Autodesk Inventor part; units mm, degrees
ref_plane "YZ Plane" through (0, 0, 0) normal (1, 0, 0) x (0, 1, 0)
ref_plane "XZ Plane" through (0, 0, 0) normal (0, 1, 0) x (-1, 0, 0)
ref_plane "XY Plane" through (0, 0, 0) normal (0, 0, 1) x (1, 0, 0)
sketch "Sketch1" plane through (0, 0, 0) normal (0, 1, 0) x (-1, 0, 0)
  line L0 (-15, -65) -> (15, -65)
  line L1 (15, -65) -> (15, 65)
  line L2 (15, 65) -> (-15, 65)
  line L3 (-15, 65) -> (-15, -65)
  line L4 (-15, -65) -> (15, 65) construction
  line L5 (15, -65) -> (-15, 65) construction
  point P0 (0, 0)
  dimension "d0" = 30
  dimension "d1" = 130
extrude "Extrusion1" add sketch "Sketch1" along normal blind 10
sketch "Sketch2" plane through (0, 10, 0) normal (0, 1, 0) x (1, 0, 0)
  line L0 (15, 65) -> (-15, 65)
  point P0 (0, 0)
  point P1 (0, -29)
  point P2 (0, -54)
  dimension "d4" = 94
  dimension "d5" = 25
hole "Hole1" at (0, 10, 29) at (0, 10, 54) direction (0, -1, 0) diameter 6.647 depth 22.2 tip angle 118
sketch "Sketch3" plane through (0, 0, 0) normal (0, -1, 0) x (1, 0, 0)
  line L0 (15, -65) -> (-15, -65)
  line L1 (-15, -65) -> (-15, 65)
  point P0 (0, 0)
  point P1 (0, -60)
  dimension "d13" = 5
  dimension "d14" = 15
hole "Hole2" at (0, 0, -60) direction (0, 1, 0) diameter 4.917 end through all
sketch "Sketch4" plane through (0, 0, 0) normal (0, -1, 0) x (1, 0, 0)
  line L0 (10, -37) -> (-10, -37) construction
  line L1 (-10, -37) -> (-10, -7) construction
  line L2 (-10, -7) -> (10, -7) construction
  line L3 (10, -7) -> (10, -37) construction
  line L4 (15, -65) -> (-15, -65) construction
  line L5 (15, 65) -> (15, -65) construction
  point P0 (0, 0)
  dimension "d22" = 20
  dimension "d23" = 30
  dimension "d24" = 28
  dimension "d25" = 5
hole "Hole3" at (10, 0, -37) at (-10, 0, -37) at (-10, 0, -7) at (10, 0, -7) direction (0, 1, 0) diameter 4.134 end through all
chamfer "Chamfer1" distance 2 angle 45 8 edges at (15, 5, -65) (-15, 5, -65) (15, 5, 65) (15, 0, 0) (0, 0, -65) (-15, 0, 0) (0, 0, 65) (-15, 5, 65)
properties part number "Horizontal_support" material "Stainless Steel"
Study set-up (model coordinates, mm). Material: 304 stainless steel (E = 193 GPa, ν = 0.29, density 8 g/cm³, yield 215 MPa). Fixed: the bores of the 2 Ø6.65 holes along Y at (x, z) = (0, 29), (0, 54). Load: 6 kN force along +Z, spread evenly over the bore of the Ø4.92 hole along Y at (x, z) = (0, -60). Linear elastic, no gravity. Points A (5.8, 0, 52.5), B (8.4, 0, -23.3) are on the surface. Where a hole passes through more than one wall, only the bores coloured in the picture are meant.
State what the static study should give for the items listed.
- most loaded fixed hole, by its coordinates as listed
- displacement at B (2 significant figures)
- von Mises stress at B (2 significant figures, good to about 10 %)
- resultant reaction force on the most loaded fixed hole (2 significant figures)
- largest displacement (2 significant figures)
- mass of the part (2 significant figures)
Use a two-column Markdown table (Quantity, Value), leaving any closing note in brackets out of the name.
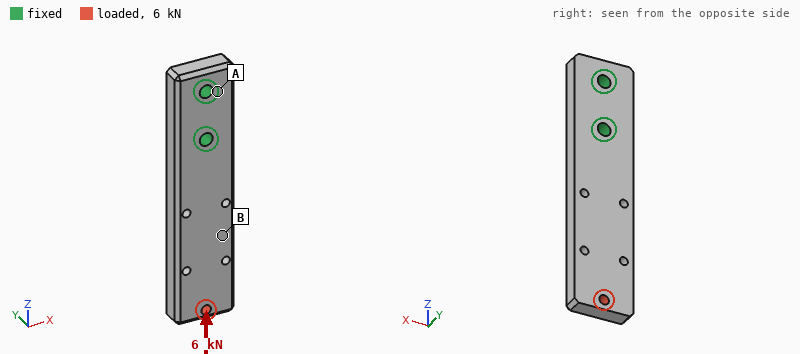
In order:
| Quantity | Value |
|---|---|
| most loaded fixed hole, by its coordinates as listed | (0, 29) |
| displacement at B | 6.5 µm |
| von Mises stress at B | 20 MPa |
| resultant reaction force on the most loaded fixed hole | 5.0 kN |
| largest displacement | 15 µm |
| mass of the part | 300 g |
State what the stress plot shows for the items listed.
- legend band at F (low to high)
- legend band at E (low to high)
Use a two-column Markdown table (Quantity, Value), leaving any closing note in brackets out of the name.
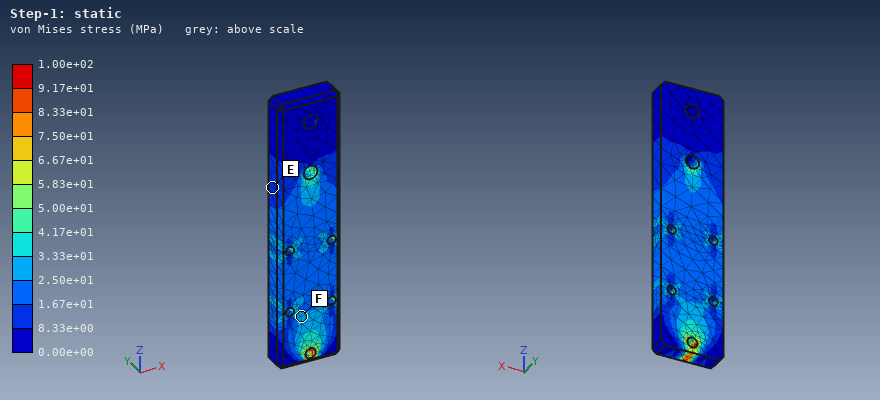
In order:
| Quantity | Value |
|---|---|
| legend band at F | 2.50e+01 to 3.33e+01 MPa |
| legend band at E | 8.33e+00 to 1.67e+01 MPa |
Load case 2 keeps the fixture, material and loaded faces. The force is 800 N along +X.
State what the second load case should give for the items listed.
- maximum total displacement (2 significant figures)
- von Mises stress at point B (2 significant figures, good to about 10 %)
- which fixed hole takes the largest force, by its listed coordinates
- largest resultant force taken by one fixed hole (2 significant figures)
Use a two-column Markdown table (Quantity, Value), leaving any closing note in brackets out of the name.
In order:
| Quantity | Value |
|---|---|
| maximum total displacement | 76 µm |
| von Mises stress at point B | 12 MPa |
| which fixed hole takes the largest force, by its listed coordinates | (0, 29) |
| largest resultant force taken by one fixed hole | 2.6 kN |
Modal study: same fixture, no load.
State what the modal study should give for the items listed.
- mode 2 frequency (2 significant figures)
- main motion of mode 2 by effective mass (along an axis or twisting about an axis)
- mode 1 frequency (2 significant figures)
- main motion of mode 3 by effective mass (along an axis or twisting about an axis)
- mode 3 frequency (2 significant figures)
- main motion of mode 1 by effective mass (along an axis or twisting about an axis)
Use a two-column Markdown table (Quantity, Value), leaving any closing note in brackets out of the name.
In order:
| Quantity | Value |
|---|---|
| mode 2 frequency | 2100 Hz |
| main motion of mode 2 by effective mass | along X |
| mode 1 frequency | 900 Hz |
| main motion of mode 3 by effective mass | twisting about Z |
| mode 3 frequency | 4700 Hz |
| main motion of mode 1 by effective mass | along Y |
